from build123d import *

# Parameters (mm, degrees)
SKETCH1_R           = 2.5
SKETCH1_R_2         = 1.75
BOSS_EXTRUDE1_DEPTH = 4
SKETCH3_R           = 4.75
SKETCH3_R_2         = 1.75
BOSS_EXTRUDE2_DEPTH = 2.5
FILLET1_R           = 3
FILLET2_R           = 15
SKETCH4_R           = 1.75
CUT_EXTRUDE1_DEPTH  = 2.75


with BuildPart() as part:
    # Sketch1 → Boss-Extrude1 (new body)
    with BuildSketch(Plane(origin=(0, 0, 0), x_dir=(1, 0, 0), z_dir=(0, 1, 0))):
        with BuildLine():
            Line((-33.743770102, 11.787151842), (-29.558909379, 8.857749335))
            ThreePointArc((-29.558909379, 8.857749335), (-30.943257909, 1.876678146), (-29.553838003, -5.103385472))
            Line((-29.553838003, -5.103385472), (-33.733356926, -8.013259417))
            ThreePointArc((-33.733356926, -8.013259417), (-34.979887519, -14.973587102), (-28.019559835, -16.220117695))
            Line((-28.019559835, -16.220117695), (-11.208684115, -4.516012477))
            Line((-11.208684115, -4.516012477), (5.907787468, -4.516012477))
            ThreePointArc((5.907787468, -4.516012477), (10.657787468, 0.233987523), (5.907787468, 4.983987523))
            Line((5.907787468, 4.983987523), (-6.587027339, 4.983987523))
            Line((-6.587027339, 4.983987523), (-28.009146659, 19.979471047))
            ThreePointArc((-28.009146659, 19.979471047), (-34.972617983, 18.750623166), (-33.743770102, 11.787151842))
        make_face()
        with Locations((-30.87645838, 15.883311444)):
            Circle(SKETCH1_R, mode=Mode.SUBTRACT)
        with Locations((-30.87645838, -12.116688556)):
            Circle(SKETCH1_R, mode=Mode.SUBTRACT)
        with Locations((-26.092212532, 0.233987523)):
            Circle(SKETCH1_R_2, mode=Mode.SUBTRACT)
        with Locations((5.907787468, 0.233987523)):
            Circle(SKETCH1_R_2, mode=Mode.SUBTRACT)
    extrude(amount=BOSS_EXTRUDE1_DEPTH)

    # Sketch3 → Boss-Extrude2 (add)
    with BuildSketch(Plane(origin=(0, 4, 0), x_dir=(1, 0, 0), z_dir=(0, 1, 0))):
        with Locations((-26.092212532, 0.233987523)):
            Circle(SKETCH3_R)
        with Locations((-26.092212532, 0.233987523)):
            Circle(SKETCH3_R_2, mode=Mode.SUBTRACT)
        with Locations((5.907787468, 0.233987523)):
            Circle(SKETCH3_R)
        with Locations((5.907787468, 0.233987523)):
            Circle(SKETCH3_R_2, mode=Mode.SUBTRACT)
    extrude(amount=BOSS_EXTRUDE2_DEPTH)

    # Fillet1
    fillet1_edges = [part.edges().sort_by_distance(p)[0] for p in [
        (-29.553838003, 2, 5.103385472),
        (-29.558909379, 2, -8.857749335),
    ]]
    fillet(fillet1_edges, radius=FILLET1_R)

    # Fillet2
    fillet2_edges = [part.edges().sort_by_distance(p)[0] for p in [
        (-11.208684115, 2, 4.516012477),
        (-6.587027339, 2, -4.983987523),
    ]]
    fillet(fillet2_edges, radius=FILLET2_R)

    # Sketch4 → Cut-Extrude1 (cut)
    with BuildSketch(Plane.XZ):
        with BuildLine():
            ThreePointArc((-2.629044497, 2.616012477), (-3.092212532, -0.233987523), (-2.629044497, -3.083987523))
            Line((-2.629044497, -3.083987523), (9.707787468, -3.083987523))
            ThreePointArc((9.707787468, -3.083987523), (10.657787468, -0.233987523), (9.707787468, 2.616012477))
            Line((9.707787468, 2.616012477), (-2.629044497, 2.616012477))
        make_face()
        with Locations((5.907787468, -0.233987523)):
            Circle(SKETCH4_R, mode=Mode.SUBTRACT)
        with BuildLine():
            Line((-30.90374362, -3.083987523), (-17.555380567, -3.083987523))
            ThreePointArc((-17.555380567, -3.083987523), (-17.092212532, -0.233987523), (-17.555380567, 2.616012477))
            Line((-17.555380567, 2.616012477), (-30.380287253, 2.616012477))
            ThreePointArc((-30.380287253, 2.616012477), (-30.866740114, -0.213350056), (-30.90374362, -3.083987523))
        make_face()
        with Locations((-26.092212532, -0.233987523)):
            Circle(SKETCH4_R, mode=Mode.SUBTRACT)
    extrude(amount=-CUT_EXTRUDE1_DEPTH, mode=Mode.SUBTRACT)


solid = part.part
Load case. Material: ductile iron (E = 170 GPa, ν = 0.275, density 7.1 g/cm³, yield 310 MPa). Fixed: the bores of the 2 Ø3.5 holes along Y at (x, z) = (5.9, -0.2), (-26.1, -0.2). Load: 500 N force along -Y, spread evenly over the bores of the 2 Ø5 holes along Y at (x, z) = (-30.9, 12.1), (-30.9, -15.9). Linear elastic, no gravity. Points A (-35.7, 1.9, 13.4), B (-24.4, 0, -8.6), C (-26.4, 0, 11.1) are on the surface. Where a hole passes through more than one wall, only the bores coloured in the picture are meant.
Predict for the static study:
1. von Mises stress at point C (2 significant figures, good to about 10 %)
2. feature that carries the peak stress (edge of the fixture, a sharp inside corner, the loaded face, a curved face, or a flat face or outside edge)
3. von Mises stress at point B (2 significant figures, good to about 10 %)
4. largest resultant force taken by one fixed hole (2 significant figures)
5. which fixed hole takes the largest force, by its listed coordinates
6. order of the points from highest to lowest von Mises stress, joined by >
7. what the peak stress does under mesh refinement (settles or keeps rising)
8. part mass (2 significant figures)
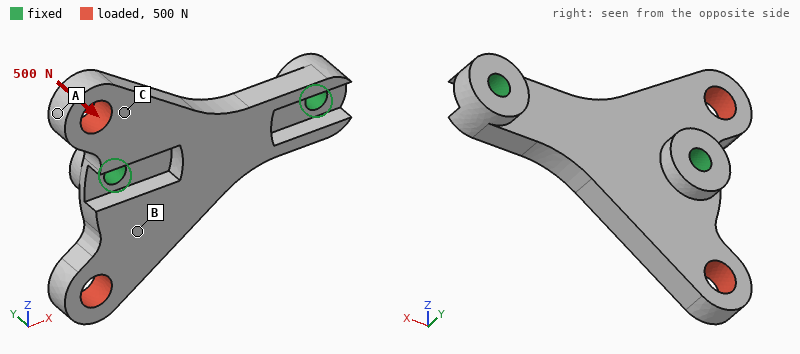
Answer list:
43 MPa
edge of the fixture
70 MPa
560 N
(-26.1, -0.2)
B > C > A
keeps rising
21 g
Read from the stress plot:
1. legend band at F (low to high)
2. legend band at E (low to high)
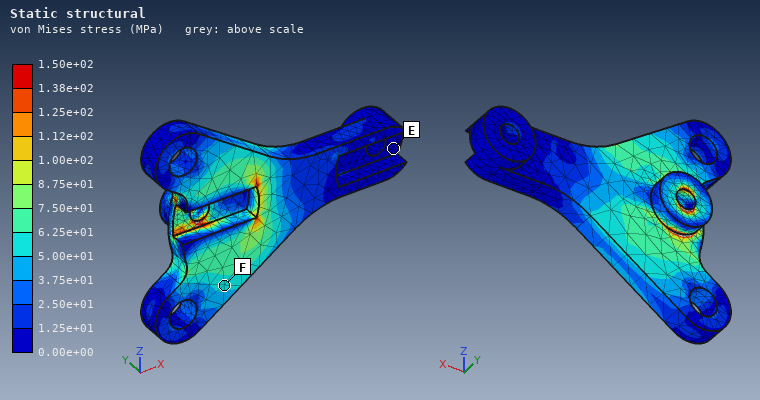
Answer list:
5.00e+01 to 6.25e+01 MPa
0.00e+00 to 1.25e+01 MPa
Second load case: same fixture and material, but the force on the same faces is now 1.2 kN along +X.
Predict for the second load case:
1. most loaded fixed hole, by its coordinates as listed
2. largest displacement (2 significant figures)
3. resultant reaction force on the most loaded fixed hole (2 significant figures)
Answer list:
(-26.1, -0.2)
17 µm
770 N
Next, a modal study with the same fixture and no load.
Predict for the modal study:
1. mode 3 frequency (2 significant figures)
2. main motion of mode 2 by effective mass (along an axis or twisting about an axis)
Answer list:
14 kHz
along Y
